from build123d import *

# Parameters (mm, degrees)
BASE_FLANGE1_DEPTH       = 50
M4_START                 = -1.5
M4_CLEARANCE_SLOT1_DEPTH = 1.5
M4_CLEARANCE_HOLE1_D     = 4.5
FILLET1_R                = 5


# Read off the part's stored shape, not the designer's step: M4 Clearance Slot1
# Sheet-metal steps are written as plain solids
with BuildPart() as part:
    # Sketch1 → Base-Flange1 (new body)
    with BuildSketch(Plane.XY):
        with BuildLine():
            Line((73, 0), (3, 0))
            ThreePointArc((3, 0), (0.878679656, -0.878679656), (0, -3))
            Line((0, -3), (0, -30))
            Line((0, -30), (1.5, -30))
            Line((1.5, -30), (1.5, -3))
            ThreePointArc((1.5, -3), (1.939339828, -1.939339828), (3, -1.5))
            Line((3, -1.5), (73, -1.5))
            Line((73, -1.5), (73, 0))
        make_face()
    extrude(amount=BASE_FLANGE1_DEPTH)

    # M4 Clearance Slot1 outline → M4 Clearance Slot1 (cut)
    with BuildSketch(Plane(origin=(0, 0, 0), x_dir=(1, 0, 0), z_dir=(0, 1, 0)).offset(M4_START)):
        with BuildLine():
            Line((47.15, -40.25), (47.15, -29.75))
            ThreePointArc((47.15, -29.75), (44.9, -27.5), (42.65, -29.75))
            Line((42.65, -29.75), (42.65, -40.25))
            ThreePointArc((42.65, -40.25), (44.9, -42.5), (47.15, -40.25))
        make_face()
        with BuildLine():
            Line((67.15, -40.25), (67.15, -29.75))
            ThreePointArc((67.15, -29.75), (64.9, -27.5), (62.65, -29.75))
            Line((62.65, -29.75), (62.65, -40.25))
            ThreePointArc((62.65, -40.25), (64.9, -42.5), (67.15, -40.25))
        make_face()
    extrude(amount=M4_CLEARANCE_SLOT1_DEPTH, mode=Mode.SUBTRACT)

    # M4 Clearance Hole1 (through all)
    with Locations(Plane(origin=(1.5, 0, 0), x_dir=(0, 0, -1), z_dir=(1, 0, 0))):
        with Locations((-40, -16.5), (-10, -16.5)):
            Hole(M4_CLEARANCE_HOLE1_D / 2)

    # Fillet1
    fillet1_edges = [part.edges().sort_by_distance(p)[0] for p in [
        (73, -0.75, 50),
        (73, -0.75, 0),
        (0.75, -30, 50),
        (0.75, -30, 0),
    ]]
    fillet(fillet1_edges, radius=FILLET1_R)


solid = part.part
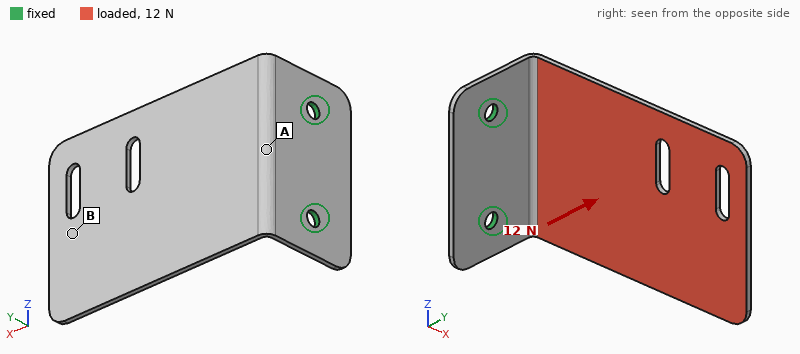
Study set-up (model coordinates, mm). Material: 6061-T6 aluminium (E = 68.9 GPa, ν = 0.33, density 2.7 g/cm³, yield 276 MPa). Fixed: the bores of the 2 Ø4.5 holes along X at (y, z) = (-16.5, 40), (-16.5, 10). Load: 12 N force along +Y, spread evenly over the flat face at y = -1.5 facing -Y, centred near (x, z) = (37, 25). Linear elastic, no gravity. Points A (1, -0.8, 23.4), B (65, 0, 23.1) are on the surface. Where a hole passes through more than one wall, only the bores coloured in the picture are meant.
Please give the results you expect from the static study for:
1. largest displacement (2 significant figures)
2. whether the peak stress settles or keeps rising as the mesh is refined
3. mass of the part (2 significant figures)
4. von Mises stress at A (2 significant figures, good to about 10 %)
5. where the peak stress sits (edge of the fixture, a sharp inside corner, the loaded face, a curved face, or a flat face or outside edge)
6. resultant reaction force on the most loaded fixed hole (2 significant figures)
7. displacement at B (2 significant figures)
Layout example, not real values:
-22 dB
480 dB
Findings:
0.99 mm
keeps rising
20 g
19 MPa
edge of the fixture
6.6 N
0.86 mm
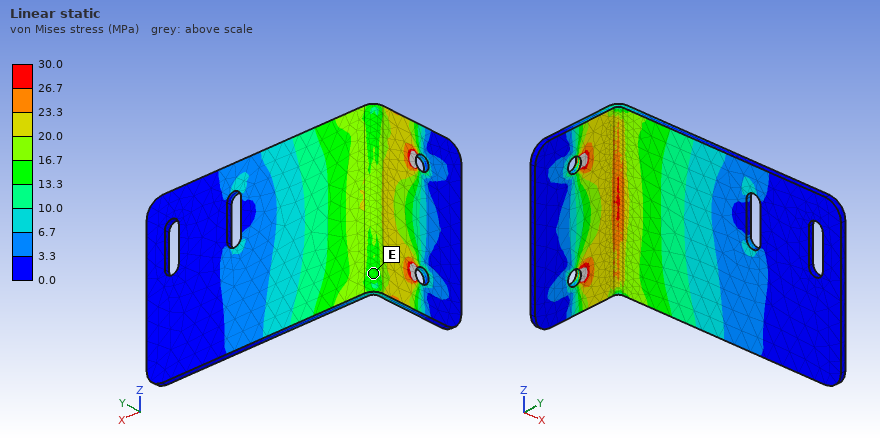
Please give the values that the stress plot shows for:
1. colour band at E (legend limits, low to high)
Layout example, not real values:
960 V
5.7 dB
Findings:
13.3 to 16.7 MPa
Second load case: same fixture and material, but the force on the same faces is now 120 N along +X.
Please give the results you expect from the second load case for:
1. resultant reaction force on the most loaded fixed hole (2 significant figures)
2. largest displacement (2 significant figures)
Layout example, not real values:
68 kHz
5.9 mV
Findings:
61 N
0.75 mm
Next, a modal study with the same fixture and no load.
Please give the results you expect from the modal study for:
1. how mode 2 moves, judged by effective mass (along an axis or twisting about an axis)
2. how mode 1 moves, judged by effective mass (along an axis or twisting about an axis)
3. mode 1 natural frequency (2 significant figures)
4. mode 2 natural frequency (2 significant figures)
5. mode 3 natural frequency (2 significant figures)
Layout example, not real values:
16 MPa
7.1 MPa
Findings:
along Z
along Y
190 Hz
570 Hz
810 Hz
